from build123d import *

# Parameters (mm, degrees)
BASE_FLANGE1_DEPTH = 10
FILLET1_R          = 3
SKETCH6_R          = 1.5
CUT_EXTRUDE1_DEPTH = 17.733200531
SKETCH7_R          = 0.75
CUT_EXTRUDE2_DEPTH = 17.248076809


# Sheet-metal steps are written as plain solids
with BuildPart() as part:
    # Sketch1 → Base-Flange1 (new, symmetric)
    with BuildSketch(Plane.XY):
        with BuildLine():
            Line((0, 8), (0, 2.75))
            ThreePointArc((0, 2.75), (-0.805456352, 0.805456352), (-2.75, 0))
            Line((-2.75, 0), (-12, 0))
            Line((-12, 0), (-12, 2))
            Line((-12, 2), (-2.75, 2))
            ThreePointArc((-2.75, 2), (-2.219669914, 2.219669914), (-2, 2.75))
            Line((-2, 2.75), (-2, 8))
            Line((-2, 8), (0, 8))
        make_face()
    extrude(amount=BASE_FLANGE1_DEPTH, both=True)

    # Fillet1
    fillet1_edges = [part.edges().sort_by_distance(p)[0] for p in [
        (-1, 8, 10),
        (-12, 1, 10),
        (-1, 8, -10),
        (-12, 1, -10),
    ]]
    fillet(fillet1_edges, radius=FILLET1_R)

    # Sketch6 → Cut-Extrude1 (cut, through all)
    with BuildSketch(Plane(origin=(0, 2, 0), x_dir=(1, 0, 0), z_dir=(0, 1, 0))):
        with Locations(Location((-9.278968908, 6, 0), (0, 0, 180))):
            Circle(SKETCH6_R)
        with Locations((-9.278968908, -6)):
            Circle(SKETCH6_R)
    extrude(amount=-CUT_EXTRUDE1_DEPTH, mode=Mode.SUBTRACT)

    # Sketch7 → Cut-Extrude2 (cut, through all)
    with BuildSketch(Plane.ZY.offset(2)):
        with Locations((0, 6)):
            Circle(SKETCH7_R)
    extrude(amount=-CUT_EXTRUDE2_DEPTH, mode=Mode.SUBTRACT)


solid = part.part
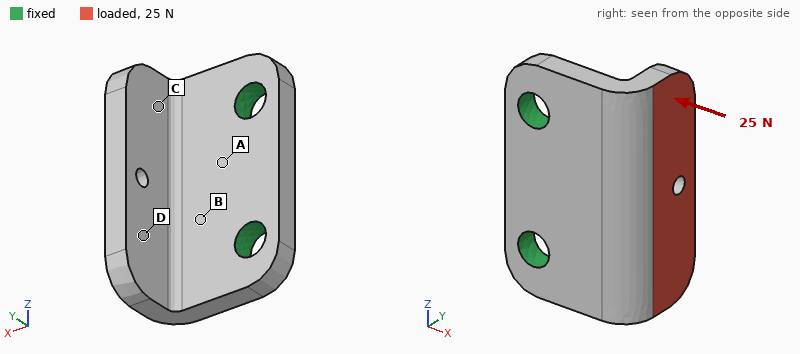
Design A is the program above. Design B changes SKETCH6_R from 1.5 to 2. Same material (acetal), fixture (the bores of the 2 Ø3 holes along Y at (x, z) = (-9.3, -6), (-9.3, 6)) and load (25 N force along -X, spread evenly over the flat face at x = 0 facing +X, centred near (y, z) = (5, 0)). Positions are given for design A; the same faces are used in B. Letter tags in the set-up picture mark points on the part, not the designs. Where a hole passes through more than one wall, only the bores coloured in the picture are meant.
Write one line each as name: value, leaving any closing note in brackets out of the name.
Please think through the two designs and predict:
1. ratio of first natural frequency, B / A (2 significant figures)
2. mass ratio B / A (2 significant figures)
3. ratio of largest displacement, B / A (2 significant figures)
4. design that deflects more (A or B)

ratio of first natural frequency, B / A: 1.1
mass ratio B / A: 0.97
ratio of largest displacement, B / A: 0.90
design that deflects more: A
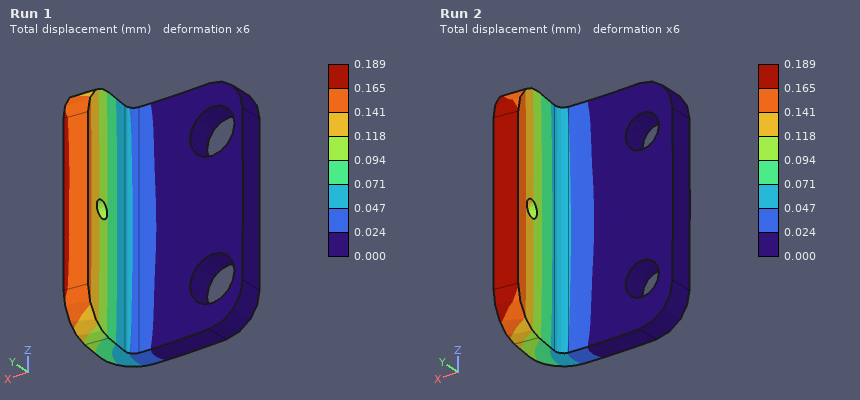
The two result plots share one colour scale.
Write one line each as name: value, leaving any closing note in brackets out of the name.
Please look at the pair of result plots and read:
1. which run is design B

which run is design B: Run 1
